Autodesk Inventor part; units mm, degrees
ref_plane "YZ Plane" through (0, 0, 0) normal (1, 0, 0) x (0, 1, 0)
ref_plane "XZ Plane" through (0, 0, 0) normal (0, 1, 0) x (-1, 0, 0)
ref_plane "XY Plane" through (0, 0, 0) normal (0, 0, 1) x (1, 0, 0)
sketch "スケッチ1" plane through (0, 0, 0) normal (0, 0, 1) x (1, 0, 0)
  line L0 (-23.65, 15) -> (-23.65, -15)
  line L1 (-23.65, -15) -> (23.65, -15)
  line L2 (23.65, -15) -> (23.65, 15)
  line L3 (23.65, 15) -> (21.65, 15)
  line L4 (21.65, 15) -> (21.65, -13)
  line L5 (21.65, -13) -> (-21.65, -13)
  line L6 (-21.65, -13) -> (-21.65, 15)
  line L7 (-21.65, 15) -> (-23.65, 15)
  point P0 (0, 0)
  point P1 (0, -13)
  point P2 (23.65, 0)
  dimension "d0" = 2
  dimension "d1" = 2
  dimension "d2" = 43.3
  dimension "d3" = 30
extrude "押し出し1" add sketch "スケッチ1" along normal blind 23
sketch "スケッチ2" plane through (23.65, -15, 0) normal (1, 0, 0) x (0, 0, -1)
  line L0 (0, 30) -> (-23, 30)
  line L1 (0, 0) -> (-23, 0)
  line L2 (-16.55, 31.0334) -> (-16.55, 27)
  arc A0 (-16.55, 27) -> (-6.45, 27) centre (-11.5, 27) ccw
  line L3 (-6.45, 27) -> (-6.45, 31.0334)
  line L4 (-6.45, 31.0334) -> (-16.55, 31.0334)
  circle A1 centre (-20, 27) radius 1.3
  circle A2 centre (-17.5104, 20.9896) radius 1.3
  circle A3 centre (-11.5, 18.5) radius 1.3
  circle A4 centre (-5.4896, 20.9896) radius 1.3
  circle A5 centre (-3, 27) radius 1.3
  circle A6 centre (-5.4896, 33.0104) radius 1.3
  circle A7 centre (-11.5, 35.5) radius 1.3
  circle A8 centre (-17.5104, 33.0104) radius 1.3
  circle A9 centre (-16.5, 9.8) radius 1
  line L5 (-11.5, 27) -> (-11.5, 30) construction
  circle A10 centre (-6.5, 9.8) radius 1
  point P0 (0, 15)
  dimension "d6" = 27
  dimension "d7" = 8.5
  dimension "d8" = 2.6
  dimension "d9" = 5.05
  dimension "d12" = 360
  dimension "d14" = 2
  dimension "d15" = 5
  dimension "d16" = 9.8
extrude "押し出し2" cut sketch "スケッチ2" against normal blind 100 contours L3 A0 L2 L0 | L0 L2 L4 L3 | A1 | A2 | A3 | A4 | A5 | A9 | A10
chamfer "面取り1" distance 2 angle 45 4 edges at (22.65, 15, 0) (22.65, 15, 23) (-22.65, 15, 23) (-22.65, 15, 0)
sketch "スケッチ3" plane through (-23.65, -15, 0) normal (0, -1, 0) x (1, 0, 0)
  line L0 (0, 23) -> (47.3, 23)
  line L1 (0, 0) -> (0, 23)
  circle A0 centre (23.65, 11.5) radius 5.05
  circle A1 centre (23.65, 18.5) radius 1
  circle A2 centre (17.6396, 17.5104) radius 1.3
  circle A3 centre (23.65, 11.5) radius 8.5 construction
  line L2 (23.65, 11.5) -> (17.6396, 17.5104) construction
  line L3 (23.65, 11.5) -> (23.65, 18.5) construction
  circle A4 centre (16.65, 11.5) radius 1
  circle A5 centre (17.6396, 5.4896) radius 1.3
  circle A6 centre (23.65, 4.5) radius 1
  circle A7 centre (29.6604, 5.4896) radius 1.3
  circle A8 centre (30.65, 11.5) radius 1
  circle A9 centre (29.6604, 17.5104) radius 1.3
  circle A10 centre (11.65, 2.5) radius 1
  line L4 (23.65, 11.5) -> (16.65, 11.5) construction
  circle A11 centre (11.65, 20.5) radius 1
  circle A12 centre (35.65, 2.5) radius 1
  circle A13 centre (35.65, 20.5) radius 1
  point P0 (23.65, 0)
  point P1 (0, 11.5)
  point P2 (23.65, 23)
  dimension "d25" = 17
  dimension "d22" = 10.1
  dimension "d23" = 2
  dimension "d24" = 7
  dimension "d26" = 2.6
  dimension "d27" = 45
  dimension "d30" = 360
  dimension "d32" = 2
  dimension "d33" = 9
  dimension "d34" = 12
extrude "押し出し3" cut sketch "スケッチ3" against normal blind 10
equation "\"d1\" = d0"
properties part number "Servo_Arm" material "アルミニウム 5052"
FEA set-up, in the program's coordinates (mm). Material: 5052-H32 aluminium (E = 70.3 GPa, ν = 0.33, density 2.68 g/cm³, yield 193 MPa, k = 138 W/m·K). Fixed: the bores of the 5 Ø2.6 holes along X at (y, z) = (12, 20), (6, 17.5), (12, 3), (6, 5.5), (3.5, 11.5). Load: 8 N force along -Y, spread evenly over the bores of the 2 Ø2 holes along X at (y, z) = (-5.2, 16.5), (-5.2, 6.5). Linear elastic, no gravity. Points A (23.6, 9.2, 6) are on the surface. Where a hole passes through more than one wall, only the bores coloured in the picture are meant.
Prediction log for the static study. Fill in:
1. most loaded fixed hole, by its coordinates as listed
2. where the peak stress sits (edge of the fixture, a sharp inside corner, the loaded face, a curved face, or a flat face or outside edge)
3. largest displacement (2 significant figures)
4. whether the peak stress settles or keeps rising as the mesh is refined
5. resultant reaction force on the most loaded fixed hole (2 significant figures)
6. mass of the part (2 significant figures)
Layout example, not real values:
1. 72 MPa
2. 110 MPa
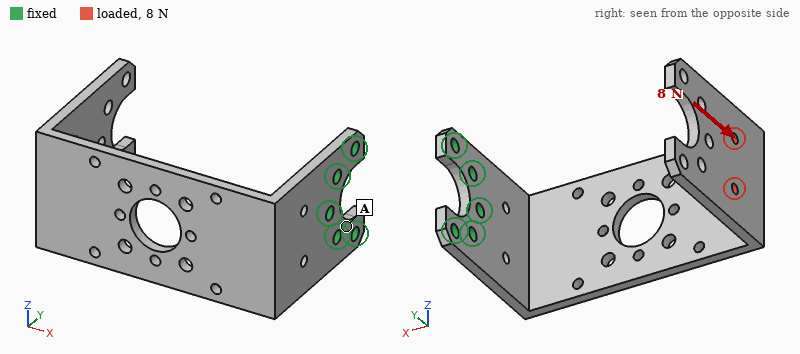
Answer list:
1. (3.5, 11.5)
2. edge of the fixture
3. 0.68 mm
4. keeps rising
5. 28 N
6. 11 g
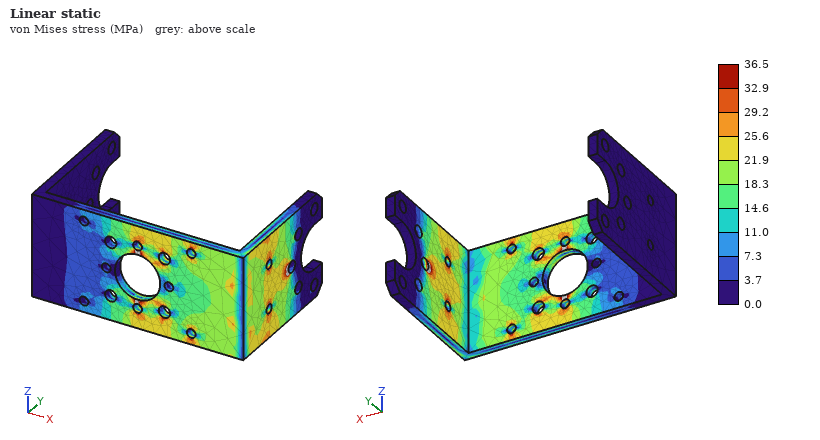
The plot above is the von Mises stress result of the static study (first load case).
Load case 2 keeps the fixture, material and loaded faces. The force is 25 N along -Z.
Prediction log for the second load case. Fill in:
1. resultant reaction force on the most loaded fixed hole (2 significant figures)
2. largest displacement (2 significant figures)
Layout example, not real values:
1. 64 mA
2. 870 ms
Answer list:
1. 72 N
2. 0.71 mm
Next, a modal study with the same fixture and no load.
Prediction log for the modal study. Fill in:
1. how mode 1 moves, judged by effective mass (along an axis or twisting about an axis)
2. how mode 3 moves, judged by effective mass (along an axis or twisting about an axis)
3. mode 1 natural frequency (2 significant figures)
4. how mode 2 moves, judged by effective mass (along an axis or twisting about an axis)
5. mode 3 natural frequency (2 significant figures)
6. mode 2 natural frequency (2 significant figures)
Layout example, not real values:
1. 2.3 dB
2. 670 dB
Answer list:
1. along Y
2. along X
3. 280 Hz
4. along Z
5. 1000 Hz
6. 500 Hz
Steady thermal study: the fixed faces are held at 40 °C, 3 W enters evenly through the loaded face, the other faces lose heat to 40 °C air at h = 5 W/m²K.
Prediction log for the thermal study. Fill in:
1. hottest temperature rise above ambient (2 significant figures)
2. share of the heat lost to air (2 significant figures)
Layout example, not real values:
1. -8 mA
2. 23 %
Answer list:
1. 37 K
2. 16 %
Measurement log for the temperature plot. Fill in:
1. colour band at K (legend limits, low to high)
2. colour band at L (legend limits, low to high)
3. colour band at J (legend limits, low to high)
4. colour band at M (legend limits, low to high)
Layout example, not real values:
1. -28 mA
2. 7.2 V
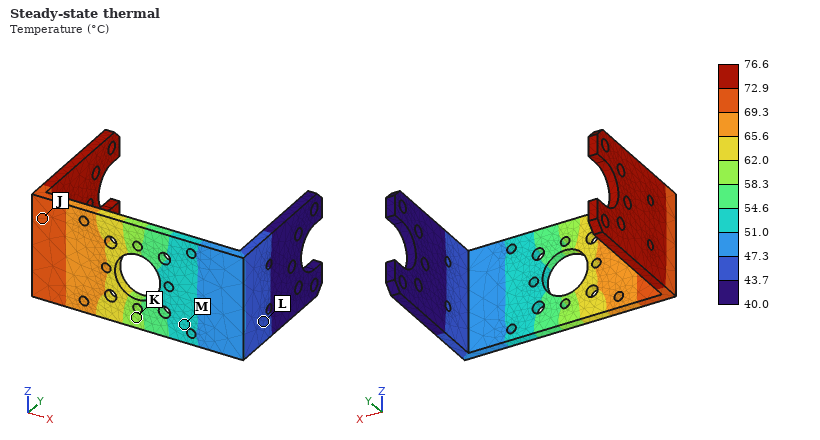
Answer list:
1. 58.3 to 62.0 °C
2. 43.7 to 47.3 °C
3. 69.3 to 72.9 °C
4. 51.0 to 54.6 °C
